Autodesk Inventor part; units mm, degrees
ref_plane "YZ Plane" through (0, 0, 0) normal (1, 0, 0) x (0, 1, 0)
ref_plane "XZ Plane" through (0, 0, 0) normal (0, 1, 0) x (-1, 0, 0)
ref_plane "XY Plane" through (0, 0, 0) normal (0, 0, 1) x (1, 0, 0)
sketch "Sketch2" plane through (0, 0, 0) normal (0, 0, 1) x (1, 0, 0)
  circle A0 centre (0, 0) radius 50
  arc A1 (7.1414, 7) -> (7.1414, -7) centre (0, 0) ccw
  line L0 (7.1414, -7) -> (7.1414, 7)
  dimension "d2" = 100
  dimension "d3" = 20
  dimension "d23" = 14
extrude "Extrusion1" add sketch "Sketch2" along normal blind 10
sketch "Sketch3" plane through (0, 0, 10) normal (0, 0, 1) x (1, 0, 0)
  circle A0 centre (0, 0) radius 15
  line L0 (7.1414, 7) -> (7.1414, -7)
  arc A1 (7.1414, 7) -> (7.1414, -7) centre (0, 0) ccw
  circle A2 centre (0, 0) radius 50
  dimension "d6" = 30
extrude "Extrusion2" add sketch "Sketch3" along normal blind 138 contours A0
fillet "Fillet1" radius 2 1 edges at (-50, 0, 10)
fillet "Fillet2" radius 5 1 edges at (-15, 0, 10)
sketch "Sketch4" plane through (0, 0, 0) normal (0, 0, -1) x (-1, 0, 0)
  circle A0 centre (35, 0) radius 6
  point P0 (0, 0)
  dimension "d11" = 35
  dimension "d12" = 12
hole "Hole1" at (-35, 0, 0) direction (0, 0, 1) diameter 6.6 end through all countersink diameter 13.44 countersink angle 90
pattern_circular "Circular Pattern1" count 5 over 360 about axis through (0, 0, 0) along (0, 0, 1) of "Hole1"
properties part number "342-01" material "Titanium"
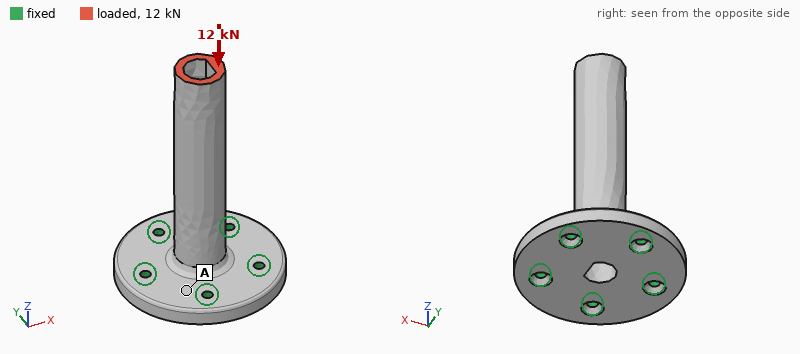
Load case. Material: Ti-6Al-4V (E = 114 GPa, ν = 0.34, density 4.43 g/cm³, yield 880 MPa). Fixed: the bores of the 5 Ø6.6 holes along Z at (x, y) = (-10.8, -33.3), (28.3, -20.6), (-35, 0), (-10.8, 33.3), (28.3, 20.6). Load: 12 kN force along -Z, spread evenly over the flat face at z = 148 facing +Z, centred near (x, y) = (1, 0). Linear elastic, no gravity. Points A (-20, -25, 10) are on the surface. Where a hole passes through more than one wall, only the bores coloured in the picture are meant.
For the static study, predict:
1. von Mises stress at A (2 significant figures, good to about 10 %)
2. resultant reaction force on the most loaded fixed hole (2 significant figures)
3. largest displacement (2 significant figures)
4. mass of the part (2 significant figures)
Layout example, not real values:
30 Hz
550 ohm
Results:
16 MPa
2.5 kN
54 µm
580 g
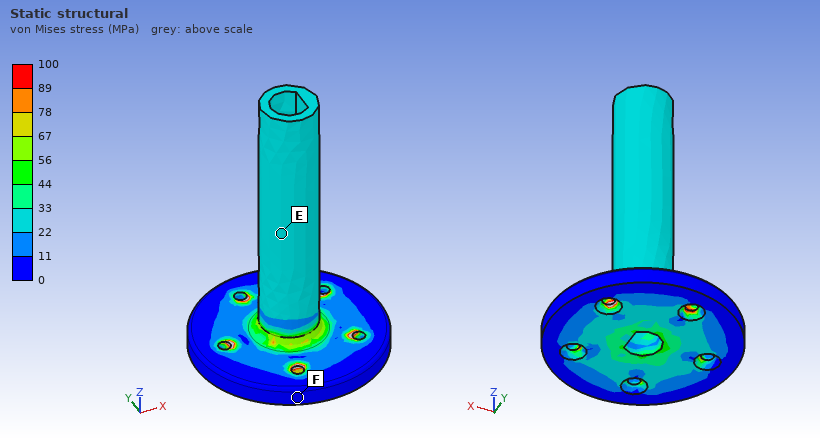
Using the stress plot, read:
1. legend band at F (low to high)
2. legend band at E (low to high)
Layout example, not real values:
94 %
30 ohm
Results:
0 to 11 MPa
22 to 33 MPa
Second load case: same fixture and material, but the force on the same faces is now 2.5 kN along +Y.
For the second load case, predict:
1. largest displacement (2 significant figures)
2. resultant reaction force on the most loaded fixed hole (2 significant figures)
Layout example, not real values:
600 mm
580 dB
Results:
0.85 mm
4.3 kN
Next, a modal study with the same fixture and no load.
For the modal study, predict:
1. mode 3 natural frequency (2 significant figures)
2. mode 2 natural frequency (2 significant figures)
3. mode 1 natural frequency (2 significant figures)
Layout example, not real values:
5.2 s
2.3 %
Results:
5500 Hz
1000 Hz
1000 Hz
